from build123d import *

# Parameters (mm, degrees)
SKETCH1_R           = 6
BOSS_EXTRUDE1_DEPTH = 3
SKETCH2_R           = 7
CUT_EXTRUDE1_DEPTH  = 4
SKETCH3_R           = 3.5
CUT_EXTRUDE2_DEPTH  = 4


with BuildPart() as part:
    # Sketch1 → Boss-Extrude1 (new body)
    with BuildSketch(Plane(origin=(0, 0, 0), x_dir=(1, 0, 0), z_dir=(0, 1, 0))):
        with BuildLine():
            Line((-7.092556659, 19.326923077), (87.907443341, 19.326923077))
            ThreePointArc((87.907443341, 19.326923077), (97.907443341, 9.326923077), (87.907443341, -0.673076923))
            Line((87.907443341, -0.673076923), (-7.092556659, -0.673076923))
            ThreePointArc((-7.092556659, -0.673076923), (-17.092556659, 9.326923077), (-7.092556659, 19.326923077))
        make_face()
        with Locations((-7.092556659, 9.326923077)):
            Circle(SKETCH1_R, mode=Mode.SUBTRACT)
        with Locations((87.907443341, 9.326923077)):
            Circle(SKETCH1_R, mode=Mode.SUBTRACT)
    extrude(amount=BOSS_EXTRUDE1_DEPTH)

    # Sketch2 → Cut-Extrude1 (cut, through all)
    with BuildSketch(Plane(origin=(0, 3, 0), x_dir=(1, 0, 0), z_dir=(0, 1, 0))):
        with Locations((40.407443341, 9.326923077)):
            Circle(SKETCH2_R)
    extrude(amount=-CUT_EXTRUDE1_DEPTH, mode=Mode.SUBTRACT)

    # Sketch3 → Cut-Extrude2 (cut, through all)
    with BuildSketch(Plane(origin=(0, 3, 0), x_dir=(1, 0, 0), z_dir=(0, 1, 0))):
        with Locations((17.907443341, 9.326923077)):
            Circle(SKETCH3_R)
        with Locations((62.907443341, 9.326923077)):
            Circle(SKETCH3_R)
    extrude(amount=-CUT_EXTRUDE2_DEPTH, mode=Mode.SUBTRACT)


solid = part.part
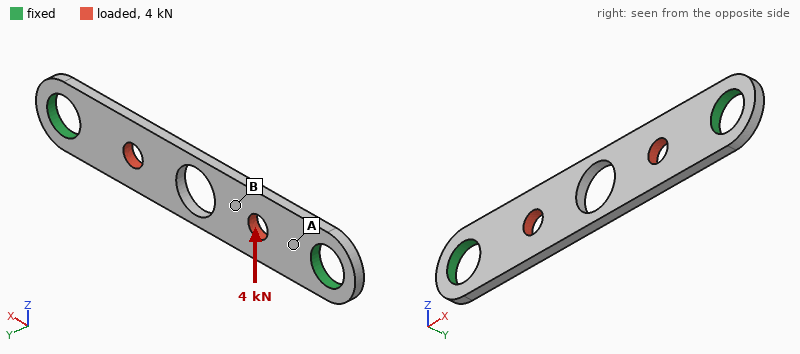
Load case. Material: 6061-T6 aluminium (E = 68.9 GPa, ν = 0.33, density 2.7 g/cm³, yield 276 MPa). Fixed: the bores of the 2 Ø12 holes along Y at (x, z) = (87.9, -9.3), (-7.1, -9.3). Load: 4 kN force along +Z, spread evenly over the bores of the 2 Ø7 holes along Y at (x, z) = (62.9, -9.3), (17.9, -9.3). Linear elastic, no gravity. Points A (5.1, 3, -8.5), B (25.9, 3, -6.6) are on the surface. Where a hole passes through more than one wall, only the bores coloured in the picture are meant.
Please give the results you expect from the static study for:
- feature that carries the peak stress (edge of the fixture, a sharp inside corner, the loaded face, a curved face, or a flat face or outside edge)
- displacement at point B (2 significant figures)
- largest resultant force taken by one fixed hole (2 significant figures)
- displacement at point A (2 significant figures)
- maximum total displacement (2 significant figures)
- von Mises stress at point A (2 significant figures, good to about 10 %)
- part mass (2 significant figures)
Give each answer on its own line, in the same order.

edge of the fixture
0.099 mm
2.0 kN
0.023 mm
0.11 mm
93 MPa
14 g
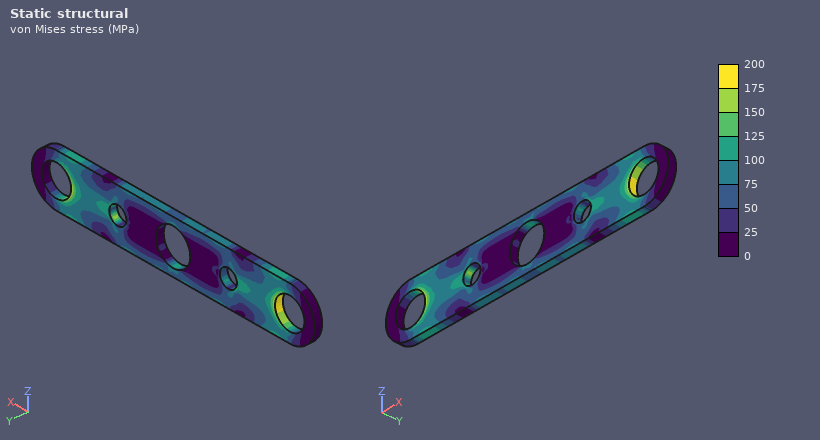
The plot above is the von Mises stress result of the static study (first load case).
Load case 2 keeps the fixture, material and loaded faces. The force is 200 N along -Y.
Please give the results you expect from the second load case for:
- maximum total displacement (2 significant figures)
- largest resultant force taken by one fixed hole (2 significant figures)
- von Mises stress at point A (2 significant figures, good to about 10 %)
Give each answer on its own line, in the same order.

0.12 mm
100 N
29 MPa
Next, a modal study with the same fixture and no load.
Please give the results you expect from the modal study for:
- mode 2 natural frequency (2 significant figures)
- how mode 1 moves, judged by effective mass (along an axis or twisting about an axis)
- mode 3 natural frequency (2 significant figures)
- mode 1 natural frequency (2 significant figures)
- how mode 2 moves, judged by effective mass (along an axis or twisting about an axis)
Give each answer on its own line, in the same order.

5400 Hz
along Y
5700 Hz
2200 Hz
twisting about X
